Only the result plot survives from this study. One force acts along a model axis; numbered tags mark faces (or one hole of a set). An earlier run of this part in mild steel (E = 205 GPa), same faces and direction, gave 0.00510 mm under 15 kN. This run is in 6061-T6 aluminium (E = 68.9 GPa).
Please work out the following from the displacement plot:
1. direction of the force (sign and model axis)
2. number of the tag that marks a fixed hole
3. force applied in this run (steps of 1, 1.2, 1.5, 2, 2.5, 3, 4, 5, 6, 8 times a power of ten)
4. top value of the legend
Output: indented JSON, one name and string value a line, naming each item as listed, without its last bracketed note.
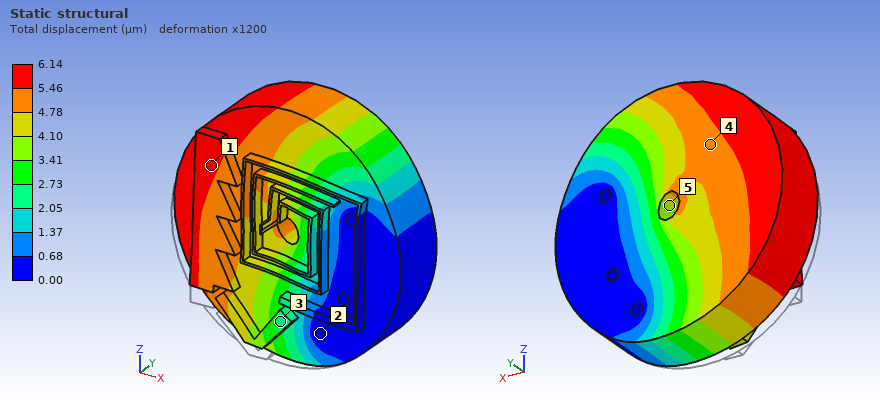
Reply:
{
  "direction of the force": "+Z",
  "number of the tag that marks a fixed hole": "2",
  "force applied in this run": "6 kN",
  "top value of the legend": "6.14 µm"
}
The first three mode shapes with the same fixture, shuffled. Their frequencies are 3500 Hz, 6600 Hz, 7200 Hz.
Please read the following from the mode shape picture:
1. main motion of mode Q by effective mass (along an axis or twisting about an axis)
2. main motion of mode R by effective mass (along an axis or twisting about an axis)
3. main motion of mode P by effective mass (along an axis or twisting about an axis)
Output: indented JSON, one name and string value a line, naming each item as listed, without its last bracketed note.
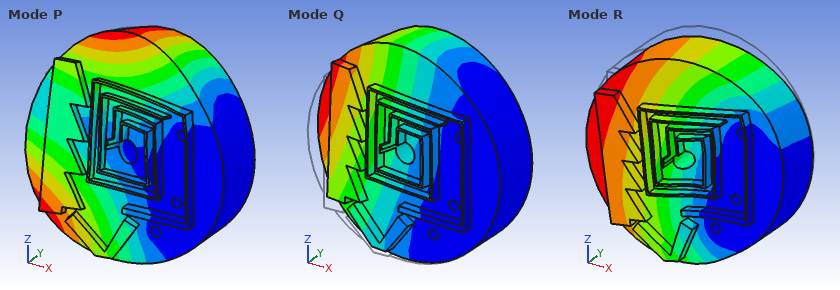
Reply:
{
  "main motion of mode Q by effective mass": "along Y",
  "main motion of mode R by effective mass": "along Z",
  "main motion of mode P by effective mass": "twisting about X"
}
